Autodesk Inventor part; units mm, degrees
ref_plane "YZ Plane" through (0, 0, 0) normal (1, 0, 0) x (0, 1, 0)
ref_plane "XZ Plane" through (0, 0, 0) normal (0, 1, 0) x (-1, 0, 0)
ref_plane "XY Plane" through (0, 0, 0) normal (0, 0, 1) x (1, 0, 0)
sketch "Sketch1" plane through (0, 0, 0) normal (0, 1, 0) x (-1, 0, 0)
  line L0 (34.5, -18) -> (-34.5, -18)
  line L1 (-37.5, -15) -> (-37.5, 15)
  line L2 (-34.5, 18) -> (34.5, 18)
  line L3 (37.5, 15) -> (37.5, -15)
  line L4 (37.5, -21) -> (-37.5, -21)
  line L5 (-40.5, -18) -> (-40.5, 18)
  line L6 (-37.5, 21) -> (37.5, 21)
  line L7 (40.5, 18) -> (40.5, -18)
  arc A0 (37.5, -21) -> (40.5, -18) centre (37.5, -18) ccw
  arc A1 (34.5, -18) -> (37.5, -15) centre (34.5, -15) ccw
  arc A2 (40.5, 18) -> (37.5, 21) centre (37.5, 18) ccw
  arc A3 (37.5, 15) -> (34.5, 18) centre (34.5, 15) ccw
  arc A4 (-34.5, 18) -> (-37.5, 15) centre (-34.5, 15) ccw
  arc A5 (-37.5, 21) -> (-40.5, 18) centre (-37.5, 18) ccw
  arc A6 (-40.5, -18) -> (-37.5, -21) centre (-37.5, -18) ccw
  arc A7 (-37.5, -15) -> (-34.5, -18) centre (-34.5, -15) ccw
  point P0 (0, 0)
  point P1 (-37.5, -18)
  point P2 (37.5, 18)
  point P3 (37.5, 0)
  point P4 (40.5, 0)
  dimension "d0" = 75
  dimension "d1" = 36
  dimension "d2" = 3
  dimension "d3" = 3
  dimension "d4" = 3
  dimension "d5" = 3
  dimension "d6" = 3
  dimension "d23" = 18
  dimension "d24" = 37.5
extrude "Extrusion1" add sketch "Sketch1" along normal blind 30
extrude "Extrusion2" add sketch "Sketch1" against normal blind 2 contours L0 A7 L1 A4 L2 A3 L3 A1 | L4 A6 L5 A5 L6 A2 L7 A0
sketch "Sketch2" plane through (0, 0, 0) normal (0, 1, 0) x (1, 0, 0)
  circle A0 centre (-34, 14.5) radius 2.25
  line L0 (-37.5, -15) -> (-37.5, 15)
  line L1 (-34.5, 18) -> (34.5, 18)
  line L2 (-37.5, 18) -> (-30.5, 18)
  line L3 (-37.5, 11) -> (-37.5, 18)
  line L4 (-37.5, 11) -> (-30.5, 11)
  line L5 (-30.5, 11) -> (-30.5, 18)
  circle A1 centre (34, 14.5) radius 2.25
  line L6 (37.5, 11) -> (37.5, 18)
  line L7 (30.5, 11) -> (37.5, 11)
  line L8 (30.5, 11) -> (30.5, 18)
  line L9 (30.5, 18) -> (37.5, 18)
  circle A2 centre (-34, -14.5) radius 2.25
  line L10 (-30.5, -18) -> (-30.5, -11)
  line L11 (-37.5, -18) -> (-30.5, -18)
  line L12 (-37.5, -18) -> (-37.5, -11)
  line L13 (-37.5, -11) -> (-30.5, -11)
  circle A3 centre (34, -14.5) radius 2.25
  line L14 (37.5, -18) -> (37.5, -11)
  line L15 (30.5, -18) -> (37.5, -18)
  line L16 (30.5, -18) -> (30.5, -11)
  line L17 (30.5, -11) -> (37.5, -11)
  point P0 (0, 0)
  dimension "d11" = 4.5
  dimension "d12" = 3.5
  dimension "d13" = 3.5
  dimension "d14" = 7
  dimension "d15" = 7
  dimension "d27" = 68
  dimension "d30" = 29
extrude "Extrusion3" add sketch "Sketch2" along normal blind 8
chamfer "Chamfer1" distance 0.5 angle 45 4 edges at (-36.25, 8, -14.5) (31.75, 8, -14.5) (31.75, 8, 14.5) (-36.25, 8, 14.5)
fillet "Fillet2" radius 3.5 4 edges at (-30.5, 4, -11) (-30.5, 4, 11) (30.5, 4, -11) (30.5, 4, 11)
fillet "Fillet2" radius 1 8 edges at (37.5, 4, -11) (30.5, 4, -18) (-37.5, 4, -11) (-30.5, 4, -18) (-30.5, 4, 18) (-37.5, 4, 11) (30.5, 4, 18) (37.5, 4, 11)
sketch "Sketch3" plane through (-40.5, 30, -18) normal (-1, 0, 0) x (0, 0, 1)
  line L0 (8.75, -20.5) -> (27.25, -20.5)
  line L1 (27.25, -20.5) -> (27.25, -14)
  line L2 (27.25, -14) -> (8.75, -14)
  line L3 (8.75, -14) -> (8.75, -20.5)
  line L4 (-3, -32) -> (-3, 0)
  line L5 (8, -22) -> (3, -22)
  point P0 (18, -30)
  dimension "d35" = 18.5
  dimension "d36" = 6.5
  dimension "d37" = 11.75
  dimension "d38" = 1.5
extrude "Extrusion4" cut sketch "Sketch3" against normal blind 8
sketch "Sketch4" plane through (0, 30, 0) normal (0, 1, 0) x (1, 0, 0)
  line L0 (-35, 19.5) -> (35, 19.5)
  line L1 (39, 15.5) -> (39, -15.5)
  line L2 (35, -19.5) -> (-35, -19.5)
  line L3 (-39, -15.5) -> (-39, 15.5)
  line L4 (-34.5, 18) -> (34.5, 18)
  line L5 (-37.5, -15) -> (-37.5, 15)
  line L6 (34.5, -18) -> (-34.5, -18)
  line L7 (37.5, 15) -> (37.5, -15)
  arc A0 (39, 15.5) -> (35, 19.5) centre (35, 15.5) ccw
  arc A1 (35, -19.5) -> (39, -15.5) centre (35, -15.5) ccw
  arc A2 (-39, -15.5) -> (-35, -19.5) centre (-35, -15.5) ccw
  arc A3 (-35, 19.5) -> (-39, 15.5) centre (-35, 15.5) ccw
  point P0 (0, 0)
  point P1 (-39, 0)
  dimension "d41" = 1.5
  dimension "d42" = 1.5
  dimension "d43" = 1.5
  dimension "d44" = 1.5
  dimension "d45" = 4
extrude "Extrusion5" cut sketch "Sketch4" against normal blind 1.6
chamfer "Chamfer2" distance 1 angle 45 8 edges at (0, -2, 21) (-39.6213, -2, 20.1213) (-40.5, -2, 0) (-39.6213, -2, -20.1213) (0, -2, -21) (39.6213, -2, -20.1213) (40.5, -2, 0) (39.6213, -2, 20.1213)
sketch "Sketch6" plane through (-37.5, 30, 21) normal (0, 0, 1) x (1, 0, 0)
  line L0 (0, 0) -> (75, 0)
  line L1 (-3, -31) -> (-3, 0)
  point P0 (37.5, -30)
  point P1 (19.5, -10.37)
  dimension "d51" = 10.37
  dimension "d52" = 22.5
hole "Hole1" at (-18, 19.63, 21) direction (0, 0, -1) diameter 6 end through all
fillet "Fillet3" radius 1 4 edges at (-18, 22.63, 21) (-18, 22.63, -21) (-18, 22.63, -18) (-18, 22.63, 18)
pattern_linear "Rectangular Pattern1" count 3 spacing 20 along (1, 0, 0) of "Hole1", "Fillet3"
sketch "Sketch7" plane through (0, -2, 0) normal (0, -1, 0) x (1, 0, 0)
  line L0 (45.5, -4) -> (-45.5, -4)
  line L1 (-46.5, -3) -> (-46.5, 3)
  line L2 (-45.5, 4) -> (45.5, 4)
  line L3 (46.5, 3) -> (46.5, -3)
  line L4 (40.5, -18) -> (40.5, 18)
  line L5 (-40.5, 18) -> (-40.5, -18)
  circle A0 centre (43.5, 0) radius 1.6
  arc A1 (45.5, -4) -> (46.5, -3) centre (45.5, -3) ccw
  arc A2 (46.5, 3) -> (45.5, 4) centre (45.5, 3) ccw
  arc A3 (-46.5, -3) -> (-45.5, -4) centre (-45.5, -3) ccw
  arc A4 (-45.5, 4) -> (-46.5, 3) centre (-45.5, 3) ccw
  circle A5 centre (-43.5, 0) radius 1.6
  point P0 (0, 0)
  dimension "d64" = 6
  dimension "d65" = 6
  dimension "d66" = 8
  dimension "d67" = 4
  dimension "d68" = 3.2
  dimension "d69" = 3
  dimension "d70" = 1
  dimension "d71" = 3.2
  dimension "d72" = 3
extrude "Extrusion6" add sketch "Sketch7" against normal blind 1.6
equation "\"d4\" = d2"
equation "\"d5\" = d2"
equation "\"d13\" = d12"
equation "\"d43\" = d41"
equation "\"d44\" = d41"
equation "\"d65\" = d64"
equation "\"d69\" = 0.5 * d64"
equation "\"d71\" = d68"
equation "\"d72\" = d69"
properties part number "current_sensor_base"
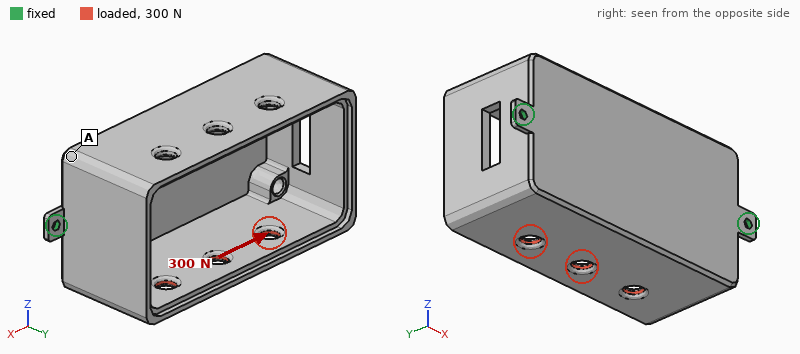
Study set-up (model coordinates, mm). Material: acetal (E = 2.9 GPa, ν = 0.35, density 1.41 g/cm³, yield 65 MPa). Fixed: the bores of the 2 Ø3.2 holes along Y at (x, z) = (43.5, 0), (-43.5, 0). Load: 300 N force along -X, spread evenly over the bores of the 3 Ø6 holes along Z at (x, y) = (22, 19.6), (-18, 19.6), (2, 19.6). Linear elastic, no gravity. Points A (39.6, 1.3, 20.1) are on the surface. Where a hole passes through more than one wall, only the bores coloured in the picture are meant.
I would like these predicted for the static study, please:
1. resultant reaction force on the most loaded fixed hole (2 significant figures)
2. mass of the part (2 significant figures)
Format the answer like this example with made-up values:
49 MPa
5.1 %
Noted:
180 N
39 g
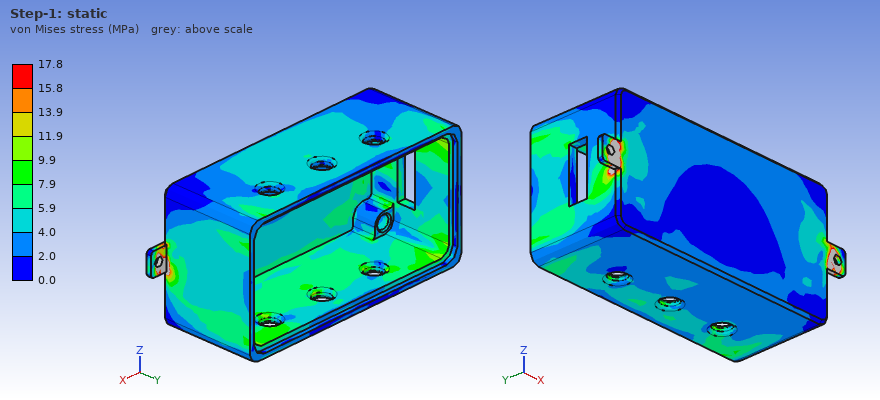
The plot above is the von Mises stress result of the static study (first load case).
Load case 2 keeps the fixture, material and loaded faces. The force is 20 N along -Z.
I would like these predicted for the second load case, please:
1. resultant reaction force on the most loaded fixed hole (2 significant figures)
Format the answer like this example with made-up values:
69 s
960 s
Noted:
11 N
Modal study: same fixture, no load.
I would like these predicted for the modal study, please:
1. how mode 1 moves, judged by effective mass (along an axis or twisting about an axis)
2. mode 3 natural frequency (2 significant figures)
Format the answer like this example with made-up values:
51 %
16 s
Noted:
along Z
900 Hz
